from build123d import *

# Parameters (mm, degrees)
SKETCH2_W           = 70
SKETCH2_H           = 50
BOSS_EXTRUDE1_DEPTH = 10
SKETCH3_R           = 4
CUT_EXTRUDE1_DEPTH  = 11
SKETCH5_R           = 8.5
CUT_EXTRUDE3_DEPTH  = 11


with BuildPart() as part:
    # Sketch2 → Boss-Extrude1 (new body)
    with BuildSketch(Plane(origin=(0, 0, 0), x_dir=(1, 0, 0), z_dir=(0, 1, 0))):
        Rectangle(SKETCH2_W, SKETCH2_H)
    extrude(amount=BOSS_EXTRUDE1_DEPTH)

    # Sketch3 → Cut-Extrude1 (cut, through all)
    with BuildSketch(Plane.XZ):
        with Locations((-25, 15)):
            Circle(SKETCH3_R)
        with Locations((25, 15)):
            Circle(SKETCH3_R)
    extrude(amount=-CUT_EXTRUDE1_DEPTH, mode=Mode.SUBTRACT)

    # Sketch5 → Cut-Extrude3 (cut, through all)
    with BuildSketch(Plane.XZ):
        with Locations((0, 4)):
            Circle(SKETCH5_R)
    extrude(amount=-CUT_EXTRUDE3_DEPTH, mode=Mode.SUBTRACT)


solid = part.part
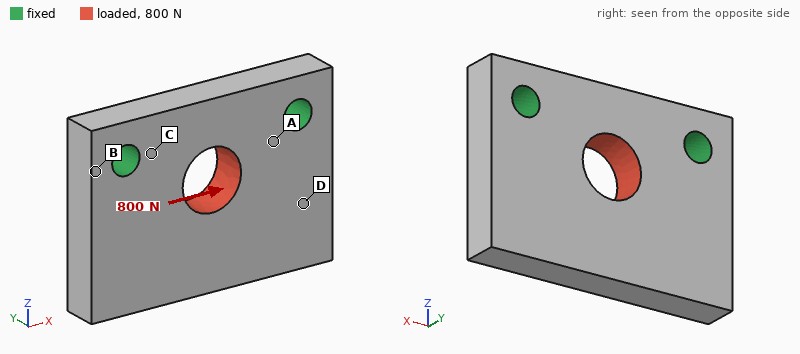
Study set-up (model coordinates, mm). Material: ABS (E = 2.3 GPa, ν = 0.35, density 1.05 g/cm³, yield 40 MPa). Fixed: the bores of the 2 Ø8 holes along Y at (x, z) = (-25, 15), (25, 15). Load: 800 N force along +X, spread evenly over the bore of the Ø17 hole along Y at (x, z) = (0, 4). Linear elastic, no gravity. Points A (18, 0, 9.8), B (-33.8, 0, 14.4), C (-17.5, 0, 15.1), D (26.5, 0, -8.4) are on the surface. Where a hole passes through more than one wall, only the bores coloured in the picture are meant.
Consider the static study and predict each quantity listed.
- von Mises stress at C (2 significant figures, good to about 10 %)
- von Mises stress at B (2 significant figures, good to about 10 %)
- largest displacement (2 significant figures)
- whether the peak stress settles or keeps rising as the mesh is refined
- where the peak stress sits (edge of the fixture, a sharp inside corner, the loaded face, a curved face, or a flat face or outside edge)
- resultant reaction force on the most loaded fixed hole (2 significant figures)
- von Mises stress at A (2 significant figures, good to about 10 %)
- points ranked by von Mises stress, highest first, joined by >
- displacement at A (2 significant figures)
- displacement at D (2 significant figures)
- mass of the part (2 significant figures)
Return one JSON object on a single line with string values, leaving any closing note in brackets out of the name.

{"von Mises stress at C": "1.8 MPa", "von Mises stress at B": "1.1 MPa", "largest displacement": "38 µm", "whether the peak stress settles or keeps rising as the mesh is refined": "keeps rising", "where the peak stress sits": "edge of the fixture", "resultant reaction force on the most loaded fixed hole": "420 N", "von Mises stress at A": "2.5 MPa", "points ranked by von Mises stress, highest first, joined by >": "A > C > B > D", "displacement at A": "8.3 µm", "displacement at D": "28 µm", "mass of the part": "33 g"}
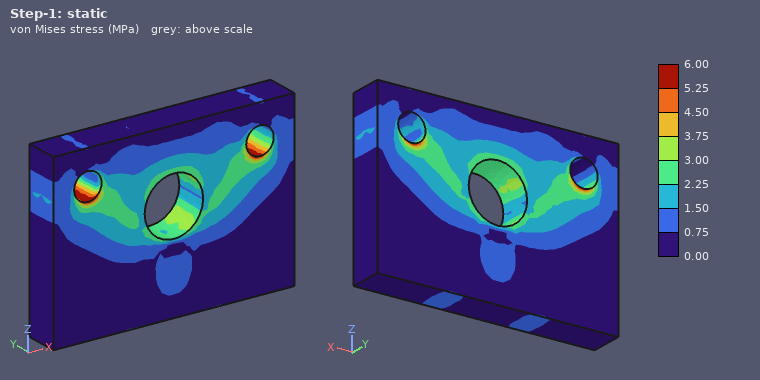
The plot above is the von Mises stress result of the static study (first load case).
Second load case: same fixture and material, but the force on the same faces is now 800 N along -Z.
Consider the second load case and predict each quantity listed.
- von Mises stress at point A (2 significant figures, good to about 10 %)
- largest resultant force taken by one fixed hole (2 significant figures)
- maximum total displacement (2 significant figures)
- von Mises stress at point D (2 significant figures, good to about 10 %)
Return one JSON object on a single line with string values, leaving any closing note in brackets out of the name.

{"von Mises stress at point A": "2.4 MPa", "largest resultant force taken by one fixed hole": "410 N", "maximum total displacement": "39 µm", "von Mises stress at point D": "0.74 MPa"}
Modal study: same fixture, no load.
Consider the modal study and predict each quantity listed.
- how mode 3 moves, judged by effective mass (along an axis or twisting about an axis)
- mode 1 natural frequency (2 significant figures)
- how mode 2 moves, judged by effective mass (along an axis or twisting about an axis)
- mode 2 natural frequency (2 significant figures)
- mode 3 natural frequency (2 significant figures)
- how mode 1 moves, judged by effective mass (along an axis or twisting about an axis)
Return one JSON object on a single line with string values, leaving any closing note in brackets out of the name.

{"how mode 3 moves, judged by effective mass": "along X", "mode 1 natural frequency": "1300 Hz", "how mode 2 moves, judged by effective mass": "twisting about Z", "mode 2 natural frequency": "2300 Hz", "mode 3 natural frequency": "3900 Hz", "how mode 1 moves, judged by effective mass": "along Y"}
